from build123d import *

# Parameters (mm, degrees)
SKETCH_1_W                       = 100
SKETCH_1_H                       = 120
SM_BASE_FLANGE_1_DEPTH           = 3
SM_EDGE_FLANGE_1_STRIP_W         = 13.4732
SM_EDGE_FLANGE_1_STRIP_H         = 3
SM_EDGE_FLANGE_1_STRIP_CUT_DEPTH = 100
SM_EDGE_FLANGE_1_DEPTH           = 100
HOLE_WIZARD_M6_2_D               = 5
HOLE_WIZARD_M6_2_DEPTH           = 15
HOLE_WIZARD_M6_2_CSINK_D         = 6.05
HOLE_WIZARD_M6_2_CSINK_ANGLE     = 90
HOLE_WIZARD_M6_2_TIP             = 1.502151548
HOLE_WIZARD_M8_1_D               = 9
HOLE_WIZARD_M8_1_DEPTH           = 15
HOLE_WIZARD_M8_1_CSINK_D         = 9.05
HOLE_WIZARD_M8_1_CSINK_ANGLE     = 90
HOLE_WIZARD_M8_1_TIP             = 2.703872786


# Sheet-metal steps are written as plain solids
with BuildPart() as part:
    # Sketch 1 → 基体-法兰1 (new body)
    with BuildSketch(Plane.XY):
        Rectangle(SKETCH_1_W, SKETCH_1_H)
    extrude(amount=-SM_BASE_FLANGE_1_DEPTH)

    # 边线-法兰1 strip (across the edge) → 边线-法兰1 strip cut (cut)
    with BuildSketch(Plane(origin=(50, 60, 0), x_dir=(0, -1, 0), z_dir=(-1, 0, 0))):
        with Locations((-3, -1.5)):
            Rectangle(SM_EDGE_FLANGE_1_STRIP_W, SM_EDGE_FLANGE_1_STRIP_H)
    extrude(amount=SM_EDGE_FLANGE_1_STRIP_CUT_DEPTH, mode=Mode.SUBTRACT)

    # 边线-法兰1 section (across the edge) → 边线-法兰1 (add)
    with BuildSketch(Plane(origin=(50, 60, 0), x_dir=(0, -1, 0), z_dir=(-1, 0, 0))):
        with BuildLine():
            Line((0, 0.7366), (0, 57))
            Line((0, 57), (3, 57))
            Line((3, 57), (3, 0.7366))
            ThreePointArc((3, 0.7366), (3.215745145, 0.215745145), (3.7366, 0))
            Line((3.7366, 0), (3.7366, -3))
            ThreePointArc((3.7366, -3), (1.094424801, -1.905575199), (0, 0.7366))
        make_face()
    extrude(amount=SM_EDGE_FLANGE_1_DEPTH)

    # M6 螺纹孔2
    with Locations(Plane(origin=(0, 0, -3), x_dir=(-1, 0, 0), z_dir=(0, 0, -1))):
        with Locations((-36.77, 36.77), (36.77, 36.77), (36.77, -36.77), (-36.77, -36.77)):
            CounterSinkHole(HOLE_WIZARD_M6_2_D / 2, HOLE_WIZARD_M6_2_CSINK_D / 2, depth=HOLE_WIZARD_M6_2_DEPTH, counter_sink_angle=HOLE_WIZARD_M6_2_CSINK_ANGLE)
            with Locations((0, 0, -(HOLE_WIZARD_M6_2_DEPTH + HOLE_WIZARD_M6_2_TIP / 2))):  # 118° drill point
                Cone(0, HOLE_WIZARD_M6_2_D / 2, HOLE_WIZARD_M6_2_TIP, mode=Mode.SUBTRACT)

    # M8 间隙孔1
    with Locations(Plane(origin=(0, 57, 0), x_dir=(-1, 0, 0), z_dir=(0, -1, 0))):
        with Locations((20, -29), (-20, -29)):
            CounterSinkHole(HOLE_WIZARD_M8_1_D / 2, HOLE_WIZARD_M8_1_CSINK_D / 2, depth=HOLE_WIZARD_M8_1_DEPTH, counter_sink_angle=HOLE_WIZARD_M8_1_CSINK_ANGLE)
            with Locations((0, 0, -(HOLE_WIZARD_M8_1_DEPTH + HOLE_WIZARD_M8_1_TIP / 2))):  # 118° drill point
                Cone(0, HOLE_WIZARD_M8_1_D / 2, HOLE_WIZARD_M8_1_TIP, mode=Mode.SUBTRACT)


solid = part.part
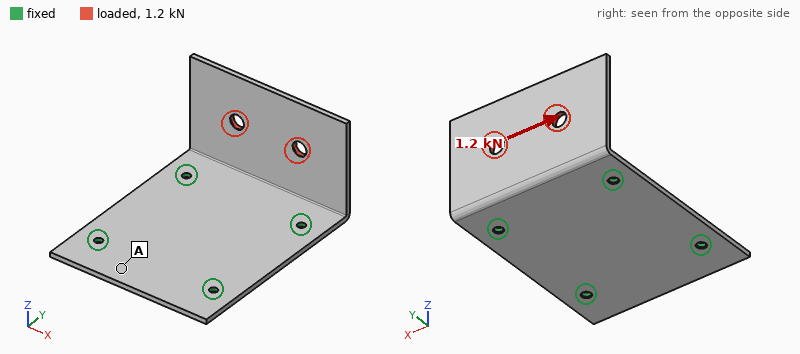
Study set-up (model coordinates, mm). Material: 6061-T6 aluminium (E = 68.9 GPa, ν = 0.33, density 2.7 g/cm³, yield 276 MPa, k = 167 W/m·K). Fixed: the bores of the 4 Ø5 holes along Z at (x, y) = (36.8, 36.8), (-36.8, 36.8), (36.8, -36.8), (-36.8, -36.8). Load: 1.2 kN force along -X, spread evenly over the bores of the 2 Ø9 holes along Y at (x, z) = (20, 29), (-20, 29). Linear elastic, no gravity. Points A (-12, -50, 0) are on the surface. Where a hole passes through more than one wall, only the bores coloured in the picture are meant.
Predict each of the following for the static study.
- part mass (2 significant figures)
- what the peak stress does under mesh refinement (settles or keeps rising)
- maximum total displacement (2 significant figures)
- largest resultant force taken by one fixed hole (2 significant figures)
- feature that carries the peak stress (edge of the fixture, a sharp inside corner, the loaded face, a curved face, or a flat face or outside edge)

140 g
keeps rising
0.56 mm
820 N
edge of the fixture
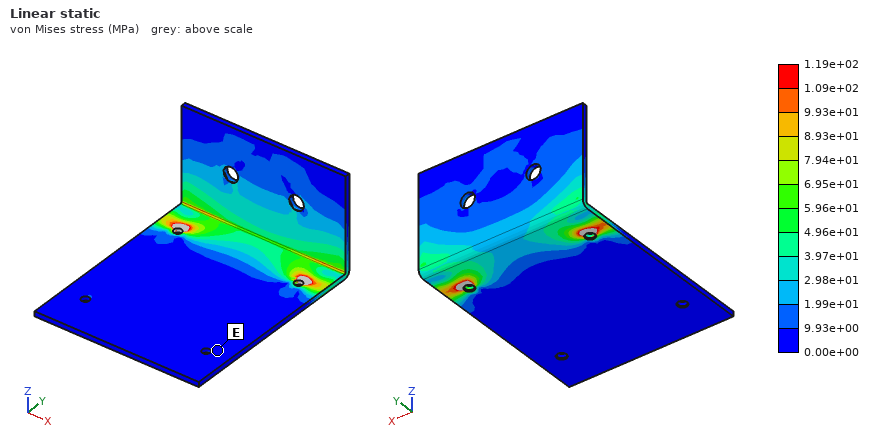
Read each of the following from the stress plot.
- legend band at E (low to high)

0.00e+00 to 9.93e+00 MPa
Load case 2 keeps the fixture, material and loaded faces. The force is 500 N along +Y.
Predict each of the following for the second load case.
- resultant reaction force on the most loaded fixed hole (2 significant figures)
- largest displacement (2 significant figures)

210 N
2.0 mm
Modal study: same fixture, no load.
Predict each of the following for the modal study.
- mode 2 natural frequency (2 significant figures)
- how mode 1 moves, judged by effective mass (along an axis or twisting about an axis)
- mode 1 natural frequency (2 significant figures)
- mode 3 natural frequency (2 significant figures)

920 Hz
along Y
450 Hz
1600 Hz
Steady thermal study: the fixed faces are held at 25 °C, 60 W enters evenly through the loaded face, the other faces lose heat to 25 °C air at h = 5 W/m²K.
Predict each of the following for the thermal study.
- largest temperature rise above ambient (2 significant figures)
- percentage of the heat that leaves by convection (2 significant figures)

81 K
7.8 %
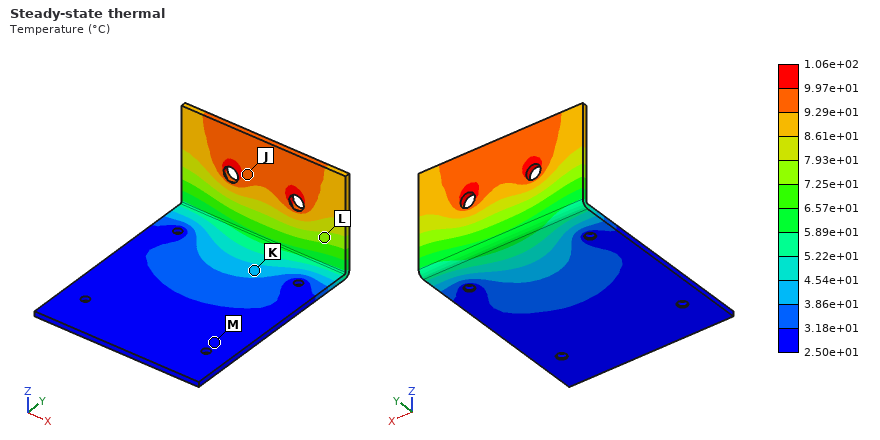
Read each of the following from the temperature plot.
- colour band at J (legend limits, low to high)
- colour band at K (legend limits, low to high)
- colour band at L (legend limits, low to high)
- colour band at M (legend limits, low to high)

9.29e+01 to 9.97e+01 °C
3.86e+01 to 4.54e+01 °C
7.25e+01 to 7.93e+01 °C
2.50e+01 to 3.18e+01 °C
